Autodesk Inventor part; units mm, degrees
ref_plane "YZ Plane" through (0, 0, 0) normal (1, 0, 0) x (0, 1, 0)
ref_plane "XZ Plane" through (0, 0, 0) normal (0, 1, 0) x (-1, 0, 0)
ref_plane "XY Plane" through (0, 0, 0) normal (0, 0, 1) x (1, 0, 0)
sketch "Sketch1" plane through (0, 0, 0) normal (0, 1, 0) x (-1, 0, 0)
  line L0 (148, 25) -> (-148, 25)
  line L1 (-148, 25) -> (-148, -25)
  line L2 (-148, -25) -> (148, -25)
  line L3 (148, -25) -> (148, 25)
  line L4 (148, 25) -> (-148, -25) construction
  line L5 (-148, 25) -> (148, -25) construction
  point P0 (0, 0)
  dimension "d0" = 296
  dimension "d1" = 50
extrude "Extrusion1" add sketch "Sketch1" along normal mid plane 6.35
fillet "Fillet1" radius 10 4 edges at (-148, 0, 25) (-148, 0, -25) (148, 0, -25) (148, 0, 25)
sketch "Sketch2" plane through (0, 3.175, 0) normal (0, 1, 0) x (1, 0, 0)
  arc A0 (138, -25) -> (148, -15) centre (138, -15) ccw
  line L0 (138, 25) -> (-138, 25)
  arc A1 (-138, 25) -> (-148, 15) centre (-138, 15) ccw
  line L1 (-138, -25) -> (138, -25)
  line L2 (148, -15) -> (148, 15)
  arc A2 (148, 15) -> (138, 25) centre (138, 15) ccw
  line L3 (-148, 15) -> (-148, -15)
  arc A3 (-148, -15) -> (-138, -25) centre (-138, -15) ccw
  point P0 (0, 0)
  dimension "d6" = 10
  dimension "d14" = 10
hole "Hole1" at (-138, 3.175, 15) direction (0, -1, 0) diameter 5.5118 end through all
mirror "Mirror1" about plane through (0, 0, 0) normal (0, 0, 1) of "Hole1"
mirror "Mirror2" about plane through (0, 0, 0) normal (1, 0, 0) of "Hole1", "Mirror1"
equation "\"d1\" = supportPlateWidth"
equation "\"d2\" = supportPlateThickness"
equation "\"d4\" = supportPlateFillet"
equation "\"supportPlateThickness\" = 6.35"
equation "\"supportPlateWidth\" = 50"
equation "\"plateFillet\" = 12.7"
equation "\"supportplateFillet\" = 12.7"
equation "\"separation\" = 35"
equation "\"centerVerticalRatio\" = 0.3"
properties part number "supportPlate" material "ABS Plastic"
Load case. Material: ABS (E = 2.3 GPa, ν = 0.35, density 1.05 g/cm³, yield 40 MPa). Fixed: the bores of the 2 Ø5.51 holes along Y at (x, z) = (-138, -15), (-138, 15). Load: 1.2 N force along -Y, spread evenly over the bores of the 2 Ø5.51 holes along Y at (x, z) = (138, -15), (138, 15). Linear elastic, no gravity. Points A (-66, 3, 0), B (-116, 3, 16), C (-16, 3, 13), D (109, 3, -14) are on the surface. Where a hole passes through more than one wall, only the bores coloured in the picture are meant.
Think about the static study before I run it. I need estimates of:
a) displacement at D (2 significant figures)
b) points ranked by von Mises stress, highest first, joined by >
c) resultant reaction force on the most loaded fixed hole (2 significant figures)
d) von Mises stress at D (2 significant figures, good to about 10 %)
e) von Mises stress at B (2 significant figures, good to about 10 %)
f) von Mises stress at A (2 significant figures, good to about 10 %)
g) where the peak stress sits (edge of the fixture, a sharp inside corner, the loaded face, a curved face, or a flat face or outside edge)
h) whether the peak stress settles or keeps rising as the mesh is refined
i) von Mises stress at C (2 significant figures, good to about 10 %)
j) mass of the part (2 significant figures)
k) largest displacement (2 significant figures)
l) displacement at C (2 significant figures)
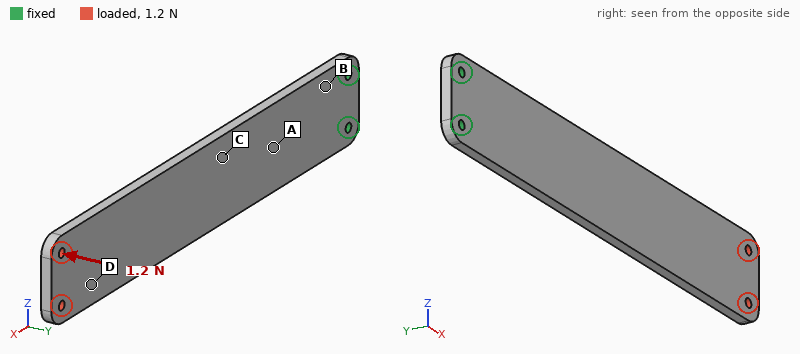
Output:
2.9 mm
B > A > C > D
0.60 N
0.11 MPa
0.89 MPa
0.73 MPa
edge of the fixture
keeps rising
0.55 MPa
97 g
3.6 mm
0.84 mm
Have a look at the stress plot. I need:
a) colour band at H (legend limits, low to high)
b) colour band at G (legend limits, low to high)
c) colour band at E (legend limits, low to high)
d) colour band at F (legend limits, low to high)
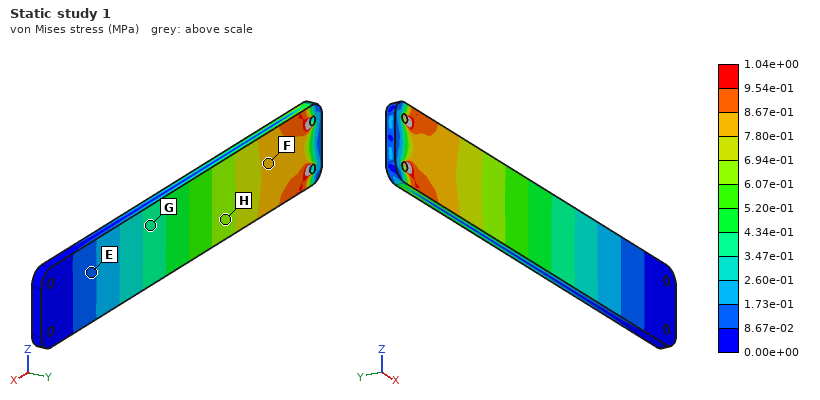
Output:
6.07e-01 to 6.94e-01 MPa
3.47e-01 to 4.34e-01 MPa
8.67e-02 to 1.73e-01 MPa
7.80e-01 to 8.67e-01 MPa
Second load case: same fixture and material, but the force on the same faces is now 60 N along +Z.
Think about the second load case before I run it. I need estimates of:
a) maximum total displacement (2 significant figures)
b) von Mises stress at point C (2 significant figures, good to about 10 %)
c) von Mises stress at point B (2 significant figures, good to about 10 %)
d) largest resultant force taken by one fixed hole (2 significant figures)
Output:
3.1 mm
1.8 MPa
3.9 MPa
510 N
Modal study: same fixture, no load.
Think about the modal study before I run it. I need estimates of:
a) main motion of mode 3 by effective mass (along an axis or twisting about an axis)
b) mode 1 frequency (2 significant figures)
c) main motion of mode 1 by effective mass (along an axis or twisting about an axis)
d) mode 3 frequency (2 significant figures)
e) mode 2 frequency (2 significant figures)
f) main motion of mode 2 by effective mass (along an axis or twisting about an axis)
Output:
along Z
19 Hz
along Y
140 Hz
120 Hz
along Y
